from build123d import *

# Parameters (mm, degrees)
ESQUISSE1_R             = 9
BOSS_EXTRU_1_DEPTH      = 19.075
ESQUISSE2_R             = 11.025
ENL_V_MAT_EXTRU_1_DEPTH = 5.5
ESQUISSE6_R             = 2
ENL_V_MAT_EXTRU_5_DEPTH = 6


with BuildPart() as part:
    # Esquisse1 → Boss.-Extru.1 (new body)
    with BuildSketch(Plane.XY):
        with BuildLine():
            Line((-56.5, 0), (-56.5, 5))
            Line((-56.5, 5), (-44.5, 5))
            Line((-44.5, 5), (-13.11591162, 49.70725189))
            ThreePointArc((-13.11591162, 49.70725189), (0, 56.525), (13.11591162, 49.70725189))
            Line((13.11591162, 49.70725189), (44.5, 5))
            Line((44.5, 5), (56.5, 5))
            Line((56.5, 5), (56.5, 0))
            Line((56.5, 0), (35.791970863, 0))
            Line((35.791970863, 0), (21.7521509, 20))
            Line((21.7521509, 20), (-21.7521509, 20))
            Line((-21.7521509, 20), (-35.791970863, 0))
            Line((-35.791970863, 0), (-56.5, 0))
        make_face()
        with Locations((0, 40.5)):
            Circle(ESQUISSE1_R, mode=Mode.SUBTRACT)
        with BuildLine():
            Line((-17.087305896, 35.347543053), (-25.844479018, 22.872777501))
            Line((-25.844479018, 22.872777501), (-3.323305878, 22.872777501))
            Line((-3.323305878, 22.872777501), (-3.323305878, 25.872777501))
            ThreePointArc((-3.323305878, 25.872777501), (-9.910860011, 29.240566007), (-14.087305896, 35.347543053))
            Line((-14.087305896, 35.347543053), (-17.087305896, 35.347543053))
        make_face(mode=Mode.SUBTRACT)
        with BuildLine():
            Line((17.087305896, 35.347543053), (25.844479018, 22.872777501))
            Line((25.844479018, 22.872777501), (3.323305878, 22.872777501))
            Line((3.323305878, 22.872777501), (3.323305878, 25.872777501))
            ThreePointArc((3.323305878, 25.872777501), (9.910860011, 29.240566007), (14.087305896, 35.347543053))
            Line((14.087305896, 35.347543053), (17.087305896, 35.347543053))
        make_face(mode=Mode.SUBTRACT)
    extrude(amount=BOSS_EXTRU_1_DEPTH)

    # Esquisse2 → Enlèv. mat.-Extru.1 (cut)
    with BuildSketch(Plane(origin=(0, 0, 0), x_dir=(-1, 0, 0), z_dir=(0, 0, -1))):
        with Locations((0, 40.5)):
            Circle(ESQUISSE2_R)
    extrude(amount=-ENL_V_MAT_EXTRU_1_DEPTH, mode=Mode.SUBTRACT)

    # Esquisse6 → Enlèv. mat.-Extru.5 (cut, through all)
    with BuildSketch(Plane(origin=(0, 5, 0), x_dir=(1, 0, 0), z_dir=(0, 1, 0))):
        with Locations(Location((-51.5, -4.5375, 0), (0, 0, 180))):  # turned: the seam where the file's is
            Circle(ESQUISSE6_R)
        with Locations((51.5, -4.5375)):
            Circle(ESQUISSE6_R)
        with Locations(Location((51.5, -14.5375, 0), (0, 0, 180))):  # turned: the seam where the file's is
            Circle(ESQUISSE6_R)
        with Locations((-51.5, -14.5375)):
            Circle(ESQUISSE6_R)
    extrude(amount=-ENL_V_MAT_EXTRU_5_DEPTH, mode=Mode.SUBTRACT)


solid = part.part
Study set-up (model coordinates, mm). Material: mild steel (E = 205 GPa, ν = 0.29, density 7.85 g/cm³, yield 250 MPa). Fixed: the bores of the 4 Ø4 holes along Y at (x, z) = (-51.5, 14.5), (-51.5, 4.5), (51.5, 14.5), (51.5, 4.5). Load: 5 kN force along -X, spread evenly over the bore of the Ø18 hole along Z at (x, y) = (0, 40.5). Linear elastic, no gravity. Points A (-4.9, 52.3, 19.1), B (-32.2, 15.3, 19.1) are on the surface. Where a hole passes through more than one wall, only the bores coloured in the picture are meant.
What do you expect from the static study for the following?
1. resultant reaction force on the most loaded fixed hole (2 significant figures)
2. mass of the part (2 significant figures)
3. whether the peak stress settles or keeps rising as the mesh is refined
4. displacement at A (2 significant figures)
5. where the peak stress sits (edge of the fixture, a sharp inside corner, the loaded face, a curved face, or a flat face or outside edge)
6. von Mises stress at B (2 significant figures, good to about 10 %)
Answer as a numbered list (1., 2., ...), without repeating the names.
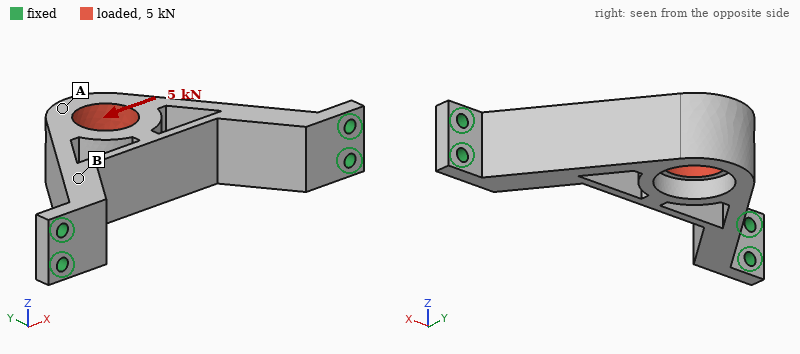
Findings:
1. 1.8 kN
2. 220 g
3. keeps rising
4. 19 µm
5. edge of the fixture
6. 29 MPa
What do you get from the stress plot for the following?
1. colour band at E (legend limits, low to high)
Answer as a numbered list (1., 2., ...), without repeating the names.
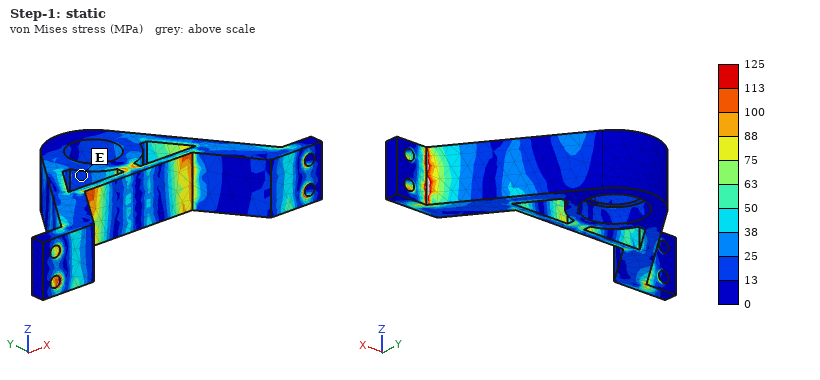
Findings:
1. 13 to 25 MPa
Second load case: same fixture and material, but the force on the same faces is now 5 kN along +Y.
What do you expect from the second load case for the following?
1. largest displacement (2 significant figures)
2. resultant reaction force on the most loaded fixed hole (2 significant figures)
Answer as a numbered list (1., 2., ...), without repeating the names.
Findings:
1. 50 µm
2. 2.2 kN
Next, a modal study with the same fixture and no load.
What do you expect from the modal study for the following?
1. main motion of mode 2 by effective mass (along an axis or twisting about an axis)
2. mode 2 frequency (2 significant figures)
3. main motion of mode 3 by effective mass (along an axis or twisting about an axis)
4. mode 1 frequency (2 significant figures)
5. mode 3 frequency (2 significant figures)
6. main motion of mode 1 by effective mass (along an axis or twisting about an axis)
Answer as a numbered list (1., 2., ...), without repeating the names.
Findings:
1. along X
2. 4600 Hz
3. along Y
4. 1800 Hz
5. 6600 Hz
6. along Z
